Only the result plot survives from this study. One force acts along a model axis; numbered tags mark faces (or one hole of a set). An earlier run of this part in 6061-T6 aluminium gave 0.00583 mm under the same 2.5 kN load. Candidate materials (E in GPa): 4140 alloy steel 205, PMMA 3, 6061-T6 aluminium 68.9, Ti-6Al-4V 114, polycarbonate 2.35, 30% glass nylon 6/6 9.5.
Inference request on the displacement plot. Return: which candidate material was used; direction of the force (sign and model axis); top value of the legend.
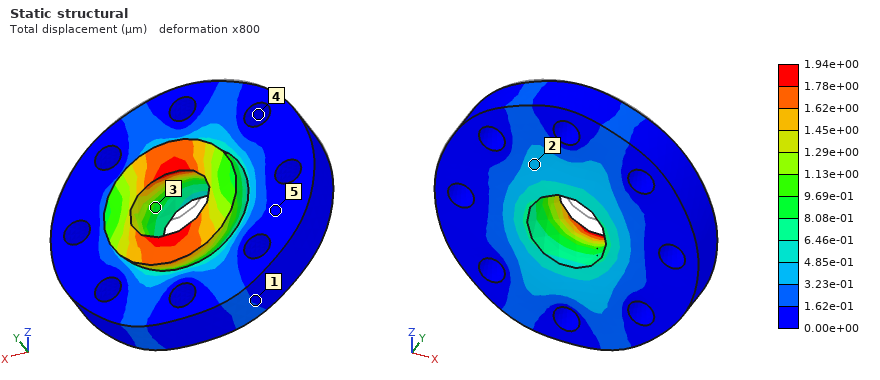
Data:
4140 alloy steel
-Z
1.94e+00 µm
